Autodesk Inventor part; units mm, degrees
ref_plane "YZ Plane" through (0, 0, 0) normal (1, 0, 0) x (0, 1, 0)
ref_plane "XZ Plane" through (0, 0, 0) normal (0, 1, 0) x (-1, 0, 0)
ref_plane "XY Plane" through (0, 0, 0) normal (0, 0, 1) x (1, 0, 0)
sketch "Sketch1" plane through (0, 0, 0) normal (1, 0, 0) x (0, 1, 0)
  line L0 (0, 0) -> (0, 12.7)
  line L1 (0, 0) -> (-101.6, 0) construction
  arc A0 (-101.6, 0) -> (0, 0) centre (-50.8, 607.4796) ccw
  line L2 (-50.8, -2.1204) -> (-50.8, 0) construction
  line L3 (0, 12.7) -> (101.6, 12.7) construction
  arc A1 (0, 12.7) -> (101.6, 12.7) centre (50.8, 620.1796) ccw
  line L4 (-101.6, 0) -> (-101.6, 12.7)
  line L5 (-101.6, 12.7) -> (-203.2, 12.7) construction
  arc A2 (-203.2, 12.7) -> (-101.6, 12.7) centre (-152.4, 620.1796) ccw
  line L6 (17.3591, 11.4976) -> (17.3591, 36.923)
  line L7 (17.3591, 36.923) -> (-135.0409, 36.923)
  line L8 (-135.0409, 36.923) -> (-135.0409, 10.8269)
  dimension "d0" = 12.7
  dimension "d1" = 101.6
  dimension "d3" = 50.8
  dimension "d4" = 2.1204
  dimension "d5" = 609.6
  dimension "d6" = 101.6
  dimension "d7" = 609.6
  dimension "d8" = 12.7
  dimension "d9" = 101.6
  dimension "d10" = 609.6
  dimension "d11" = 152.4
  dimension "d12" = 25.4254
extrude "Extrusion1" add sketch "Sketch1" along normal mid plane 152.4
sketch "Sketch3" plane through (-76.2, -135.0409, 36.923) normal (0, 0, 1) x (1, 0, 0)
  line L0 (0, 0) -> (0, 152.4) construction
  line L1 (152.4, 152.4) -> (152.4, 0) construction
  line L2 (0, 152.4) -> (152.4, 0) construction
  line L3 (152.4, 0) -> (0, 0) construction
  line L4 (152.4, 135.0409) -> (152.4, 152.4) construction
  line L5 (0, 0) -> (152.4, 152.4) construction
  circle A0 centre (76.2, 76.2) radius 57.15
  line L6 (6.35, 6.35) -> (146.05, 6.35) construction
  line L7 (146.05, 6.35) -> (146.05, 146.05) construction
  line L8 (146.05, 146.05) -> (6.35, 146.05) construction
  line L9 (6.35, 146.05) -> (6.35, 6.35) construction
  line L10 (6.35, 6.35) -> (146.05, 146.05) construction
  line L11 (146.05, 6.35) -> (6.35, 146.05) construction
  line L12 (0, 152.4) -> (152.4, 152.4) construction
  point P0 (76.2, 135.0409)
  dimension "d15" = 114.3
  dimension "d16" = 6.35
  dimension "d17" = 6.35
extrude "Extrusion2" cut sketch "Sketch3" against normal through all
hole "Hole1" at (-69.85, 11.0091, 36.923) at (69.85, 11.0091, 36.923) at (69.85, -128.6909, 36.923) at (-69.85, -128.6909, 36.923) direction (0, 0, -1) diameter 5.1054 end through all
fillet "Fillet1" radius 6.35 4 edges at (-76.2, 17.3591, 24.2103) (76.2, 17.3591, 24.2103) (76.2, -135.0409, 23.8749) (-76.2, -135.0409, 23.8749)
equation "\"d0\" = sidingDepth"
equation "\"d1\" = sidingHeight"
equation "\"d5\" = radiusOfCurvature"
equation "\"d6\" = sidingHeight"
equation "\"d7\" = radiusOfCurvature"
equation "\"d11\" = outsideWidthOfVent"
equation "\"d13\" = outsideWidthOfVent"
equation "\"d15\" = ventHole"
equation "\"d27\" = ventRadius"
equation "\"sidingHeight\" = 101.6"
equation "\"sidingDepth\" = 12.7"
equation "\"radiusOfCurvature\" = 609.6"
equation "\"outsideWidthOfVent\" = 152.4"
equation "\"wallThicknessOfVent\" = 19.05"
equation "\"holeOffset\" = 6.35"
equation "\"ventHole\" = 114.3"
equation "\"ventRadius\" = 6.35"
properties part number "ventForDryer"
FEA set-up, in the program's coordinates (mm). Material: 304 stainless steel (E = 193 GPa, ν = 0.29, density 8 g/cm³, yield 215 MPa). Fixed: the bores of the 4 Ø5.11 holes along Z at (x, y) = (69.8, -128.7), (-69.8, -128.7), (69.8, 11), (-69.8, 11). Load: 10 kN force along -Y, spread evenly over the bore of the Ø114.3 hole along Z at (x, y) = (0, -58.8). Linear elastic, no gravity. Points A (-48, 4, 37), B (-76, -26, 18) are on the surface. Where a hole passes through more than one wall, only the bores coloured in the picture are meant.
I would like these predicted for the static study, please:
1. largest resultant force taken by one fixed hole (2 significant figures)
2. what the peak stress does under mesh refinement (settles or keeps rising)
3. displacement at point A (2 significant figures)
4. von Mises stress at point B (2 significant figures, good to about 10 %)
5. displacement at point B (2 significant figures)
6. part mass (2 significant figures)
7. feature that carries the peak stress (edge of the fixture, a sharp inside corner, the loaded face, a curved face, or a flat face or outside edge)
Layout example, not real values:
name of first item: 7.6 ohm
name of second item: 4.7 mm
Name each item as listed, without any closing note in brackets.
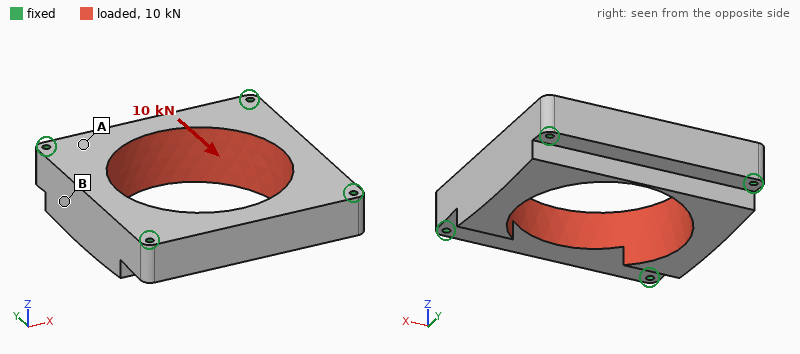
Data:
largest resultant force taken by one fixed hole: 2.7 kN
what the peak stress does under mesh refinement: keeps rising
displacement at point A: 1.8 µm
von Mises stress at point B: 6.1 MPa
displacement at point B: 1.9 µm
part mass: 3.2 kg
feature that carries the peak stress: edge of the fixture
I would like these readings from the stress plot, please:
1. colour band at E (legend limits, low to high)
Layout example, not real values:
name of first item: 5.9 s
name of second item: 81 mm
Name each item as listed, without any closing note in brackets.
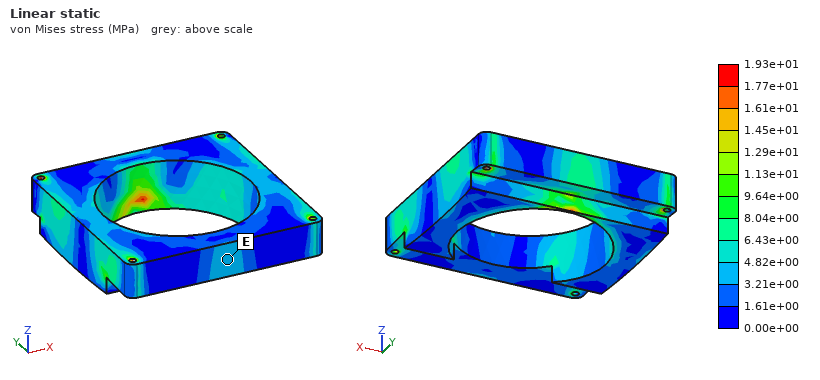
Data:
colour band at E: 3.21e+00 to 4.82e+00 MPa
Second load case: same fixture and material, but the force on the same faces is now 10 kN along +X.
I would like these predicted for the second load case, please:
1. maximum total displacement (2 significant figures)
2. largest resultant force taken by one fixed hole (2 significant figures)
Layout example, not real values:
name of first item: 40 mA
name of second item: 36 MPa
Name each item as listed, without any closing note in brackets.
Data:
maximum total displacement: 5.2 µm
largest resultant force taken by one fixed hole: 2.9 kN
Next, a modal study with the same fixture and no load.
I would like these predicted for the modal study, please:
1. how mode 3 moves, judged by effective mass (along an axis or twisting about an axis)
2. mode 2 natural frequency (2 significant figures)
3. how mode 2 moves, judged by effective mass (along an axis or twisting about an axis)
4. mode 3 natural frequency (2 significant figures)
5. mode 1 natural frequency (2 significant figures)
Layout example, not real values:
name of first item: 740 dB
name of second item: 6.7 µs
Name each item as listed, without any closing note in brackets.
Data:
how mode 3 moves, judged by effective mass: along X
mode 2 natural frequency: 4400 Hz
how mode 2 moves, judged by effective mass: along Z
mode 3 natural frequency: 5200 Hz
mode 1 natural frequency: 3100 Hz
